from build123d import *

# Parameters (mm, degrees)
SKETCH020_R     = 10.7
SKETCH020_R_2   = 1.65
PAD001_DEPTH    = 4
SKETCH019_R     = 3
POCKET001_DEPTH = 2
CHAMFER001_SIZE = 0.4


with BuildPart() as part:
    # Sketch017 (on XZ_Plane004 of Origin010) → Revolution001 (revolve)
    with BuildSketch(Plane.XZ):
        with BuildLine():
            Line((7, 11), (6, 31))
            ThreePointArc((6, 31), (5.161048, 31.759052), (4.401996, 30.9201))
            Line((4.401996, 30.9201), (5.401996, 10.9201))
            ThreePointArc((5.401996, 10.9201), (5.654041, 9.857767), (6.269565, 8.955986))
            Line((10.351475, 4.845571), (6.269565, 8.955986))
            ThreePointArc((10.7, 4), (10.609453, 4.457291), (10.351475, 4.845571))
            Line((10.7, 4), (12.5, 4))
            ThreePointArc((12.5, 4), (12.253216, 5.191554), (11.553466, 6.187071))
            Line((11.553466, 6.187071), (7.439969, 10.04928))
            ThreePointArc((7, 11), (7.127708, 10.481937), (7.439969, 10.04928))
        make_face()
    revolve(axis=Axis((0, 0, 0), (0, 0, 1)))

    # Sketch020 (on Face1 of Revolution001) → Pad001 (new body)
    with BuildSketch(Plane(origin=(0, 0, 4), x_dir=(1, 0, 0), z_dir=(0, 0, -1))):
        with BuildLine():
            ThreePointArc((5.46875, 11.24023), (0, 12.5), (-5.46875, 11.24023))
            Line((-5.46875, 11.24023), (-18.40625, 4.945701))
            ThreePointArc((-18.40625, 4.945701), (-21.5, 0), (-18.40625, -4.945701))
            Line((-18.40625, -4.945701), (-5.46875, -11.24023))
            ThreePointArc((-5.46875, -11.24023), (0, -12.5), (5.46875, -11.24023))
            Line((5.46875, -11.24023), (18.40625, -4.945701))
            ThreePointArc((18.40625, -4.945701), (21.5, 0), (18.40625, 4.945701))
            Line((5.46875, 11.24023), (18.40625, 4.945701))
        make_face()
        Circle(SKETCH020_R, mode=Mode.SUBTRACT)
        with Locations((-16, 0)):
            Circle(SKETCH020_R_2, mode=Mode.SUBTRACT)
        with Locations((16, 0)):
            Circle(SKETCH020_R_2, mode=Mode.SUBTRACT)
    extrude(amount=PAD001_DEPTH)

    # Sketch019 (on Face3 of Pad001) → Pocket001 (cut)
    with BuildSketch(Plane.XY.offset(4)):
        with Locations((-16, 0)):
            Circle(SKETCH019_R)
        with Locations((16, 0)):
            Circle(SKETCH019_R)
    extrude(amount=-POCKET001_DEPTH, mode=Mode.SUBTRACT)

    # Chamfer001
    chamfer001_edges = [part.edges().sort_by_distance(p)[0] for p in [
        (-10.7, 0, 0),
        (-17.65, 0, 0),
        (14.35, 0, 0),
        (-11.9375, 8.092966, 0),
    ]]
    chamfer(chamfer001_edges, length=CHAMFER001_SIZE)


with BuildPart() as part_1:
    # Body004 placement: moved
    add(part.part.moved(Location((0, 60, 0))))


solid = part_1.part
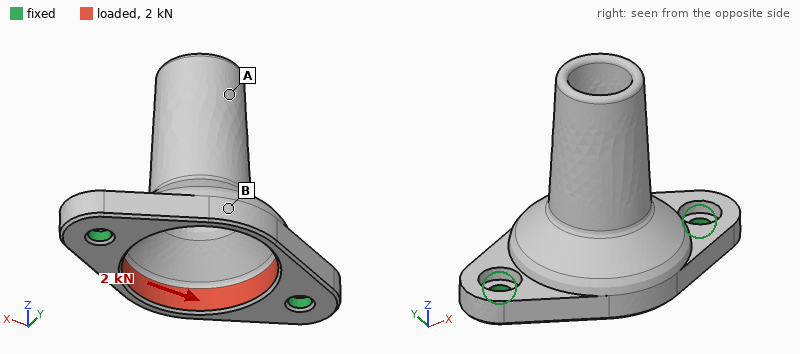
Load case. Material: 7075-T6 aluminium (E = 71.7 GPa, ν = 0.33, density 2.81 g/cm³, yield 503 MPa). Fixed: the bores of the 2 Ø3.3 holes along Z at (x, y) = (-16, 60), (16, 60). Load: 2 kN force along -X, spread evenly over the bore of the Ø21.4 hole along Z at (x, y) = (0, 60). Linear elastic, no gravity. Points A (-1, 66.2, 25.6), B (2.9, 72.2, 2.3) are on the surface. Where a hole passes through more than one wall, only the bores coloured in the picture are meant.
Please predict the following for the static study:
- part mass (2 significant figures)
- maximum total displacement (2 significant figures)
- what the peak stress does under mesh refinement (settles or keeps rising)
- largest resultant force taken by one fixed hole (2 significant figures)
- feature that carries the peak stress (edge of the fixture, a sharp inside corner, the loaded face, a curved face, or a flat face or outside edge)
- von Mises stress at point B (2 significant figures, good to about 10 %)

9.4 g
22 µm
keeps rising
1.0 kN
edge of the fixture
36 MPa
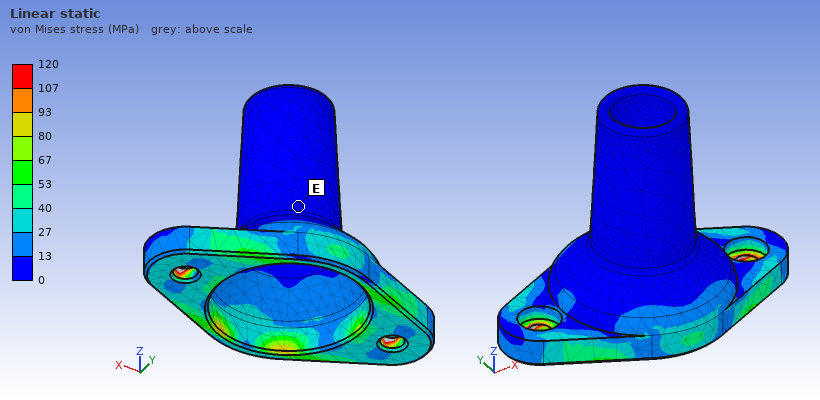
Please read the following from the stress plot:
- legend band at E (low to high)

0 to 13 MPa
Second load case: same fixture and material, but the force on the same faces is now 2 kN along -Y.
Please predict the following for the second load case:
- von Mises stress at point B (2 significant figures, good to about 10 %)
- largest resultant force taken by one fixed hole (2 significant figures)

36 MPa
1.0 kN
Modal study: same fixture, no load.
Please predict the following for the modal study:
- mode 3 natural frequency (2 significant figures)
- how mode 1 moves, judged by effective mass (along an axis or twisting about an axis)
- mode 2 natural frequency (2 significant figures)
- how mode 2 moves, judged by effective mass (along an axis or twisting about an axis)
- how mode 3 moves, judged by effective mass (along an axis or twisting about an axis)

15 kHz
along Y
12 kHz
along X
along Z
